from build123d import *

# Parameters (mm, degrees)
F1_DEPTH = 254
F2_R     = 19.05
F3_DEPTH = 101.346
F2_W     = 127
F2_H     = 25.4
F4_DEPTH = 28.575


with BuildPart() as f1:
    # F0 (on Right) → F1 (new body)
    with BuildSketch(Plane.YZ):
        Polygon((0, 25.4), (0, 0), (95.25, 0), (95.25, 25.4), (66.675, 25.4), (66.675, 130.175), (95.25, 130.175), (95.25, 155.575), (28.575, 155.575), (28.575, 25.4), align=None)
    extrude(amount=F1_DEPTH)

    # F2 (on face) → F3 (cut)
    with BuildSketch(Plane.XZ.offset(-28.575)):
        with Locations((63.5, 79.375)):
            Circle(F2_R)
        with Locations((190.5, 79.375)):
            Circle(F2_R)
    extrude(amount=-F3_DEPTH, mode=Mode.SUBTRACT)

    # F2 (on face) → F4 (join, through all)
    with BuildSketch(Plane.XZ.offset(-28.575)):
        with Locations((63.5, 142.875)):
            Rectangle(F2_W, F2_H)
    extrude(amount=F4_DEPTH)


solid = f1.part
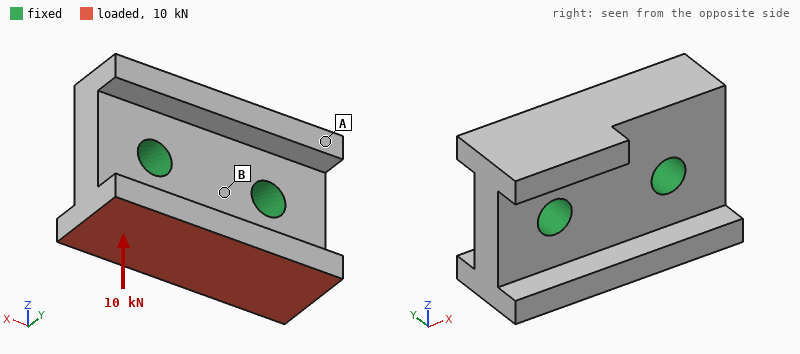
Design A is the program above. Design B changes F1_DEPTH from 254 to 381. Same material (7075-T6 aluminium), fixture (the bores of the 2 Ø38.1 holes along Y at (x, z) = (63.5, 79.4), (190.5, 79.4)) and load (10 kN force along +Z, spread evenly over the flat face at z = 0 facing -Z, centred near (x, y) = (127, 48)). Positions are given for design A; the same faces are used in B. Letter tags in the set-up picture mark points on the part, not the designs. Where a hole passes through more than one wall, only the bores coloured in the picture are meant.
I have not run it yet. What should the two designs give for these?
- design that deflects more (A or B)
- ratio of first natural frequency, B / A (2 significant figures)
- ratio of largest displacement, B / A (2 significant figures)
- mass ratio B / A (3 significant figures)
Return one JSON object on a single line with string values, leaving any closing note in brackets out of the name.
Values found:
{"design that deflects more": "B", "ratio of first natural frequency, B / A": "0.38", "ratio of largest displacement, B / A": "5.0", "mass ratio B / A": "1.50"}
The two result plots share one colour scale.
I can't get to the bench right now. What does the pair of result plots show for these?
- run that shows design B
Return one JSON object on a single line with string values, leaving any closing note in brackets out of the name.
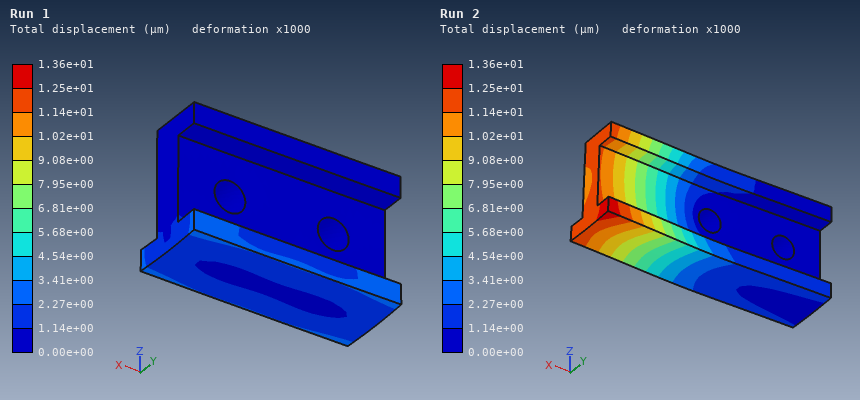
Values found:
{"run that shows design B": "Run 2"}
